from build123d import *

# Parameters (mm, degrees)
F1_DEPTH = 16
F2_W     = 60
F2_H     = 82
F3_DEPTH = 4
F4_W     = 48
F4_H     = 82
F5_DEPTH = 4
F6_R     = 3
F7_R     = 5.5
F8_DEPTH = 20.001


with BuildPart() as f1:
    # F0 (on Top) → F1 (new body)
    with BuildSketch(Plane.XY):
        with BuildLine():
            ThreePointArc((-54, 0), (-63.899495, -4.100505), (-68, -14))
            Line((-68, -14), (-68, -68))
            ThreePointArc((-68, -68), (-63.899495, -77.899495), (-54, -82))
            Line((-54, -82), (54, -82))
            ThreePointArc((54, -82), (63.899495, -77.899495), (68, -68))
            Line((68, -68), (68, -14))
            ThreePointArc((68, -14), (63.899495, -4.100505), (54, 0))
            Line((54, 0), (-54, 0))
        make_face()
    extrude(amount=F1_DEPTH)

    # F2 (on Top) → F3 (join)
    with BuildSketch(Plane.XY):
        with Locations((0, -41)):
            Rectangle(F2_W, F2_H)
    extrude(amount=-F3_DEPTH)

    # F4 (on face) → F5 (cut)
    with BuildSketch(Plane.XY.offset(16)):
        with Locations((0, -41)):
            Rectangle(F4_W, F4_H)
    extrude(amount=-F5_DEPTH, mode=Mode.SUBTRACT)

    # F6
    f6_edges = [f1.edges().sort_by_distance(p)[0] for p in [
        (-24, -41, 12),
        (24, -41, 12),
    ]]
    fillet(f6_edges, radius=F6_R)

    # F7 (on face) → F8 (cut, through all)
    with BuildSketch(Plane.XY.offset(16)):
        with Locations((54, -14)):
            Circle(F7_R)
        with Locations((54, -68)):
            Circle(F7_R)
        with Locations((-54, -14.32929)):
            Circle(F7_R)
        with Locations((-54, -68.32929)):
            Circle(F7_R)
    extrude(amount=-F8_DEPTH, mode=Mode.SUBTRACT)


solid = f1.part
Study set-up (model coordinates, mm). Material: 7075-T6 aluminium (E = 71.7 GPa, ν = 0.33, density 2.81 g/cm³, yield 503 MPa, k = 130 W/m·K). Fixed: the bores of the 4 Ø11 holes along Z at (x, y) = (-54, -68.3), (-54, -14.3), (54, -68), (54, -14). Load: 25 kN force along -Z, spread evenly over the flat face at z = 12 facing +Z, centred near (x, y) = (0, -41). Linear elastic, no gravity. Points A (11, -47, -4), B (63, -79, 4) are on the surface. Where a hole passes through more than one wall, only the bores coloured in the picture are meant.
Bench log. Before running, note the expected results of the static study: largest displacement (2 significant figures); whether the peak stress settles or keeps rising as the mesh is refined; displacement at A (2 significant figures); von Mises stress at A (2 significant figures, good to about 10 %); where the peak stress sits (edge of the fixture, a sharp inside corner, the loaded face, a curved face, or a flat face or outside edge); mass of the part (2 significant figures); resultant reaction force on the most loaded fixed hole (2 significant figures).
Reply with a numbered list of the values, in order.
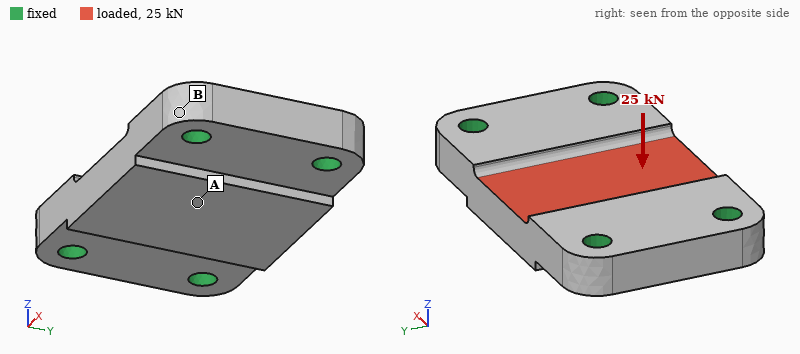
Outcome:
1. 84 µm
2. keeps rising
3. 71 µm
4. 50 MPa
5. edge of the fixture
6. 490 g
7. 8.3 kN
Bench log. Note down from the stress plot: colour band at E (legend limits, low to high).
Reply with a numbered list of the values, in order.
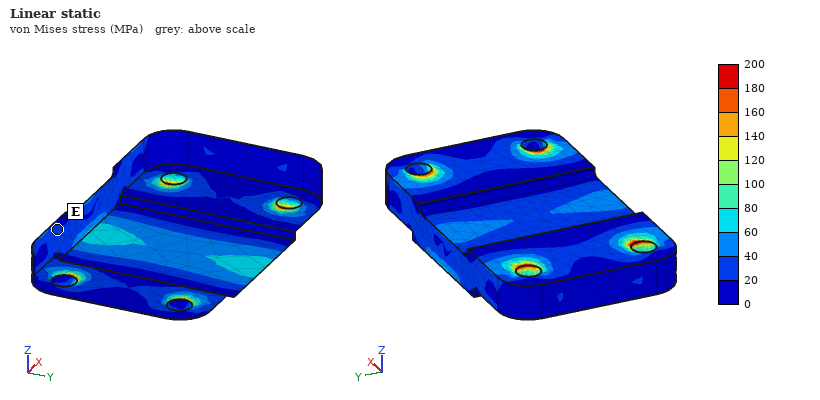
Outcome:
1. 20 to 40 MPa
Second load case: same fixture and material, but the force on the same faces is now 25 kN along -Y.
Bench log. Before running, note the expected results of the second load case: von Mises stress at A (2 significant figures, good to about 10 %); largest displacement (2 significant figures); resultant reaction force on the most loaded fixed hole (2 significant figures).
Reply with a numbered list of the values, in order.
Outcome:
1. 7.5 MPa
2. 34 µm
3. 7.5 kN
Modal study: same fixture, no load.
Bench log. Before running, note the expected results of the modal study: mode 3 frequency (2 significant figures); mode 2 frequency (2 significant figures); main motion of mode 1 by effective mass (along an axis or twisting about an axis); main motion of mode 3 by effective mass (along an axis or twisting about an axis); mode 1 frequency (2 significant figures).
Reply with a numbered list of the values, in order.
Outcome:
1. 12 kHz
2. 8400 Hz
3. along Z
4. along Y
5. 6500 Hz
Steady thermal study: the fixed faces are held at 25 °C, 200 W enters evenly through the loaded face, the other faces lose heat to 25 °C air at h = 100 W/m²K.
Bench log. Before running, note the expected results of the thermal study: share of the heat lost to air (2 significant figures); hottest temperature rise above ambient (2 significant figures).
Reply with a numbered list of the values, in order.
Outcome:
1. 12 %
2. 26 K
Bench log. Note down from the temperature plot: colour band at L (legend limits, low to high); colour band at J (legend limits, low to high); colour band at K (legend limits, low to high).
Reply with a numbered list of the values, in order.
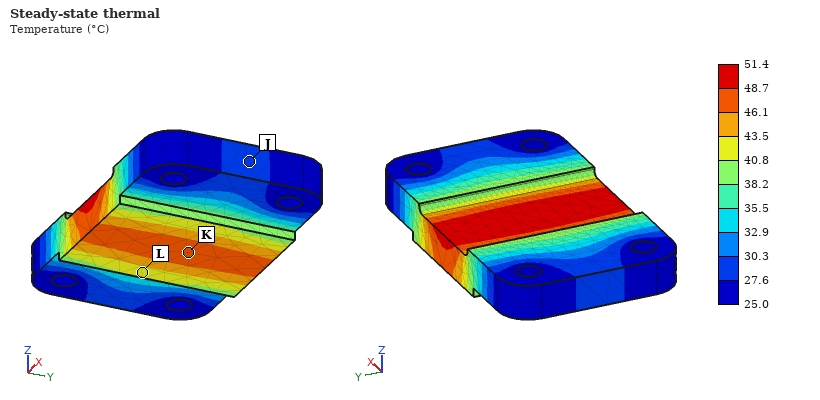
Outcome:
1. 40.8 to 43.5 °C
2. 27.6 to 30.3 °C
3. 46.1 to 48.7 °C
